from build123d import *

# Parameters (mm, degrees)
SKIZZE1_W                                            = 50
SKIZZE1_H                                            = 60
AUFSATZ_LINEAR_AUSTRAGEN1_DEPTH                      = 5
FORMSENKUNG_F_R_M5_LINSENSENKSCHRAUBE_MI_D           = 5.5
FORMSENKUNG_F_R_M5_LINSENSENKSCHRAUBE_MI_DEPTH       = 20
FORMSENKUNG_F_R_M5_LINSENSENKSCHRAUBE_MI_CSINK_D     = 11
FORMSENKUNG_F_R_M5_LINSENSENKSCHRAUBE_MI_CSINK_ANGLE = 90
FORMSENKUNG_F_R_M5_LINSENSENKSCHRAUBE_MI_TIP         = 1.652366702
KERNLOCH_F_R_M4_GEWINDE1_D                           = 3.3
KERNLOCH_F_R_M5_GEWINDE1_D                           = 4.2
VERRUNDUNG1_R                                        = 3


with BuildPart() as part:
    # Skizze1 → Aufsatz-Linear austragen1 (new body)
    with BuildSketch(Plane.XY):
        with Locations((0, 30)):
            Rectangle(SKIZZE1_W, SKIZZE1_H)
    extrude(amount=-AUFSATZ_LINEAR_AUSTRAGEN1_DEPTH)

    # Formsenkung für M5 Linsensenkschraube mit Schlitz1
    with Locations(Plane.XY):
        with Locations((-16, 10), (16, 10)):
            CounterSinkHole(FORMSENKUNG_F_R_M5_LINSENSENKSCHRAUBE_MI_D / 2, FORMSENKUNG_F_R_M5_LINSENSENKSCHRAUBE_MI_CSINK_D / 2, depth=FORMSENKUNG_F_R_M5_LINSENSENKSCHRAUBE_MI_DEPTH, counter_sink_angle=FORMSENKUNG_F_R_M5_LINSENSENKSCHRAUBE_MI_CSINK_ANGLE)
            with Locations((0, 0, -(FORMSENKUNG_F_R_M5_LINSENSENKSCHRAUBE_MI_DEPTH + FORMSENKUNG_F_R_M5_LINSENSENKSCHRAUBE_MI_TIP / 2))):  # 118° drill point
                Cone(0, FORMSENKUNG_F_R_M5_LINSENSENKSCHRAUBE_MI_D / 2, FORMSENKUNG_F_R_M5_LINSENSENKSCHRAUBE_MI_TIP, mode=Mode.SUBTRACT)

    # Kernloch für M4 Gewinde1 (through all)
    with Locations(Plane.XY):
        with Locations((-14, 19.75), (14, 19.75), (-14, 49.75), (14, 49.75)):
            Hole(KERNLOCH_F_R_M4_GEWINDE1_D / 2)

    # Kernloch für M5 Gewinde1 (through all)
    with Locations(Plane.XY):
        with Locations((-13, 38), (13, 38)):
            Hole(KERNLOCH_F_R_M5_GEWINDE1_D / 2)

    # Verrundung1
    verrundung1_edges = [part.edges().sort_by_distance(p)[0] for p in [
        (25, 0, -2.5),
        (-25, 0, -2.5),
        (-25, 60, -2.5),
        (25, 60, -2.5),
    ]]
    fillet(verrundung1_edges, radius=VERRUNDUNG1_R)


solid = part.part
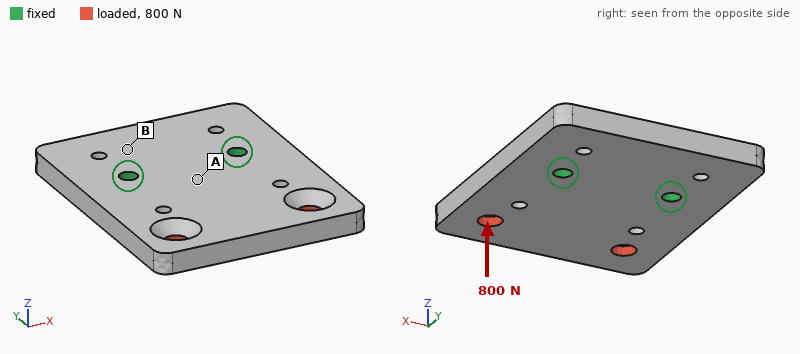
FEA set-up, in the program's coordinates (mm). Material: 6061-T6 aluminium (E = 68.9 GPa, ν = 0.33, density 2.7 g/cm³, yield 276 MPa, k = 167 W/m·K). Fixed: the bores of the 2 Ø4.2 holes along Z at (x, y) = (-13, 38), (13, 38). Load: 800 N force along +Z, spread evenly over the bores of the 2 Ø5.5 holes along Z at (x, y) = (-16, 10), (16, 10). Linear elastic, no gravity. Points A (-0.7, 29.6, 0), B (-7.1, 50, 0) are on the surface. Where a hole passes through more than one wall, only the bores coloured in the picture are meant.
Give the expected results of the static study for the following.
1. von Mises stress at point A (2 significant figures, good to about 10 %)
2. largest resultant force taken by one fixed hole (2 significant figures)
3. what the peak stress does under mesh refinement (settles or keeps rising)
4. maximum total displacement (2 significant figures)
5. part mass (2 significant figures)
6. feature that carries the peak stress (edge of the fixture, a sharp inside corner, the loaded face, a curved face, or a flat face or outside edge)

62 MPa
400 N
keeps rising
0.27 mm
38 g
edge of the fixture
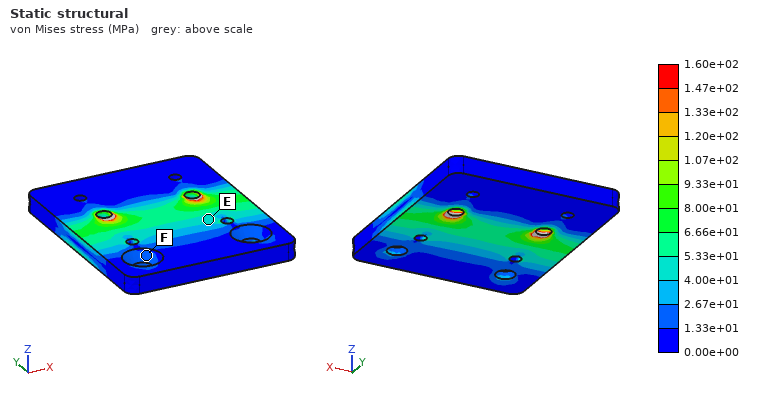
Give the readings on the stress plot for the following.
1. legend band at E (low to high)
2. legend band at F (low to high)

4.00e+01 to 5.33e+01 MPa
1.33e+01 to 2.67e+01 MPa
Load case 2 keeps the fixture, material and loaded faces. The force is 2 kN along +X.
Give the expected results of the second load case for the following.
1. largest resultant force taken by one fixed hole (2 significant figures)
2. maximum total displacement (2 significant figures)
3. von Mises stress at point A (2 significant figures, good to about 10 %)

2.2 kN
39 µm
17 MPa
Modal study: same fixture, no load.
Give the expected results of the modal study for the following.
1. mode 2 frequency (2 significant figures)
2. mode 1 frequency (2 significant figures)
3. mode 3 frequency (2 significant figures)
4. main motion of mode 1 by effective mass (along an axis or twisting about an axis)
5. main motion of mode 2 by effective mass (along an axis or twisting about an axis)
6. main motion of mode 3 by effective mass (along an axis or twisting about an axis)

5300 Hz
2800 Hz
7800 Hz
along Z
twisting about Y
along Z
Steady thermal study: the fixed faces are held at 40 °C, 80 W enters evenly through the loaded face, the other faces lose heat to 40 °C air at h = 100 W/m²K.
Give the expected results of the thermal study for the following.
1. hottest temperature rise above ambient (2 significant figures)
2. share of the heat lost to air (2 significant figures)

66 K
20 %
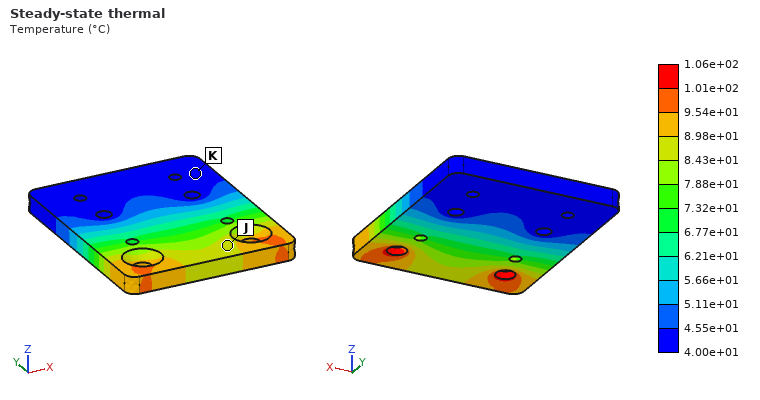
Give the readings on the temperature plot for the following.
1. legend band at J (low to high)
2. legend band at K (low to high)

8.43e+01 to 8.98e+01 °C
4.00e+01 to 4.55e+01 °C
